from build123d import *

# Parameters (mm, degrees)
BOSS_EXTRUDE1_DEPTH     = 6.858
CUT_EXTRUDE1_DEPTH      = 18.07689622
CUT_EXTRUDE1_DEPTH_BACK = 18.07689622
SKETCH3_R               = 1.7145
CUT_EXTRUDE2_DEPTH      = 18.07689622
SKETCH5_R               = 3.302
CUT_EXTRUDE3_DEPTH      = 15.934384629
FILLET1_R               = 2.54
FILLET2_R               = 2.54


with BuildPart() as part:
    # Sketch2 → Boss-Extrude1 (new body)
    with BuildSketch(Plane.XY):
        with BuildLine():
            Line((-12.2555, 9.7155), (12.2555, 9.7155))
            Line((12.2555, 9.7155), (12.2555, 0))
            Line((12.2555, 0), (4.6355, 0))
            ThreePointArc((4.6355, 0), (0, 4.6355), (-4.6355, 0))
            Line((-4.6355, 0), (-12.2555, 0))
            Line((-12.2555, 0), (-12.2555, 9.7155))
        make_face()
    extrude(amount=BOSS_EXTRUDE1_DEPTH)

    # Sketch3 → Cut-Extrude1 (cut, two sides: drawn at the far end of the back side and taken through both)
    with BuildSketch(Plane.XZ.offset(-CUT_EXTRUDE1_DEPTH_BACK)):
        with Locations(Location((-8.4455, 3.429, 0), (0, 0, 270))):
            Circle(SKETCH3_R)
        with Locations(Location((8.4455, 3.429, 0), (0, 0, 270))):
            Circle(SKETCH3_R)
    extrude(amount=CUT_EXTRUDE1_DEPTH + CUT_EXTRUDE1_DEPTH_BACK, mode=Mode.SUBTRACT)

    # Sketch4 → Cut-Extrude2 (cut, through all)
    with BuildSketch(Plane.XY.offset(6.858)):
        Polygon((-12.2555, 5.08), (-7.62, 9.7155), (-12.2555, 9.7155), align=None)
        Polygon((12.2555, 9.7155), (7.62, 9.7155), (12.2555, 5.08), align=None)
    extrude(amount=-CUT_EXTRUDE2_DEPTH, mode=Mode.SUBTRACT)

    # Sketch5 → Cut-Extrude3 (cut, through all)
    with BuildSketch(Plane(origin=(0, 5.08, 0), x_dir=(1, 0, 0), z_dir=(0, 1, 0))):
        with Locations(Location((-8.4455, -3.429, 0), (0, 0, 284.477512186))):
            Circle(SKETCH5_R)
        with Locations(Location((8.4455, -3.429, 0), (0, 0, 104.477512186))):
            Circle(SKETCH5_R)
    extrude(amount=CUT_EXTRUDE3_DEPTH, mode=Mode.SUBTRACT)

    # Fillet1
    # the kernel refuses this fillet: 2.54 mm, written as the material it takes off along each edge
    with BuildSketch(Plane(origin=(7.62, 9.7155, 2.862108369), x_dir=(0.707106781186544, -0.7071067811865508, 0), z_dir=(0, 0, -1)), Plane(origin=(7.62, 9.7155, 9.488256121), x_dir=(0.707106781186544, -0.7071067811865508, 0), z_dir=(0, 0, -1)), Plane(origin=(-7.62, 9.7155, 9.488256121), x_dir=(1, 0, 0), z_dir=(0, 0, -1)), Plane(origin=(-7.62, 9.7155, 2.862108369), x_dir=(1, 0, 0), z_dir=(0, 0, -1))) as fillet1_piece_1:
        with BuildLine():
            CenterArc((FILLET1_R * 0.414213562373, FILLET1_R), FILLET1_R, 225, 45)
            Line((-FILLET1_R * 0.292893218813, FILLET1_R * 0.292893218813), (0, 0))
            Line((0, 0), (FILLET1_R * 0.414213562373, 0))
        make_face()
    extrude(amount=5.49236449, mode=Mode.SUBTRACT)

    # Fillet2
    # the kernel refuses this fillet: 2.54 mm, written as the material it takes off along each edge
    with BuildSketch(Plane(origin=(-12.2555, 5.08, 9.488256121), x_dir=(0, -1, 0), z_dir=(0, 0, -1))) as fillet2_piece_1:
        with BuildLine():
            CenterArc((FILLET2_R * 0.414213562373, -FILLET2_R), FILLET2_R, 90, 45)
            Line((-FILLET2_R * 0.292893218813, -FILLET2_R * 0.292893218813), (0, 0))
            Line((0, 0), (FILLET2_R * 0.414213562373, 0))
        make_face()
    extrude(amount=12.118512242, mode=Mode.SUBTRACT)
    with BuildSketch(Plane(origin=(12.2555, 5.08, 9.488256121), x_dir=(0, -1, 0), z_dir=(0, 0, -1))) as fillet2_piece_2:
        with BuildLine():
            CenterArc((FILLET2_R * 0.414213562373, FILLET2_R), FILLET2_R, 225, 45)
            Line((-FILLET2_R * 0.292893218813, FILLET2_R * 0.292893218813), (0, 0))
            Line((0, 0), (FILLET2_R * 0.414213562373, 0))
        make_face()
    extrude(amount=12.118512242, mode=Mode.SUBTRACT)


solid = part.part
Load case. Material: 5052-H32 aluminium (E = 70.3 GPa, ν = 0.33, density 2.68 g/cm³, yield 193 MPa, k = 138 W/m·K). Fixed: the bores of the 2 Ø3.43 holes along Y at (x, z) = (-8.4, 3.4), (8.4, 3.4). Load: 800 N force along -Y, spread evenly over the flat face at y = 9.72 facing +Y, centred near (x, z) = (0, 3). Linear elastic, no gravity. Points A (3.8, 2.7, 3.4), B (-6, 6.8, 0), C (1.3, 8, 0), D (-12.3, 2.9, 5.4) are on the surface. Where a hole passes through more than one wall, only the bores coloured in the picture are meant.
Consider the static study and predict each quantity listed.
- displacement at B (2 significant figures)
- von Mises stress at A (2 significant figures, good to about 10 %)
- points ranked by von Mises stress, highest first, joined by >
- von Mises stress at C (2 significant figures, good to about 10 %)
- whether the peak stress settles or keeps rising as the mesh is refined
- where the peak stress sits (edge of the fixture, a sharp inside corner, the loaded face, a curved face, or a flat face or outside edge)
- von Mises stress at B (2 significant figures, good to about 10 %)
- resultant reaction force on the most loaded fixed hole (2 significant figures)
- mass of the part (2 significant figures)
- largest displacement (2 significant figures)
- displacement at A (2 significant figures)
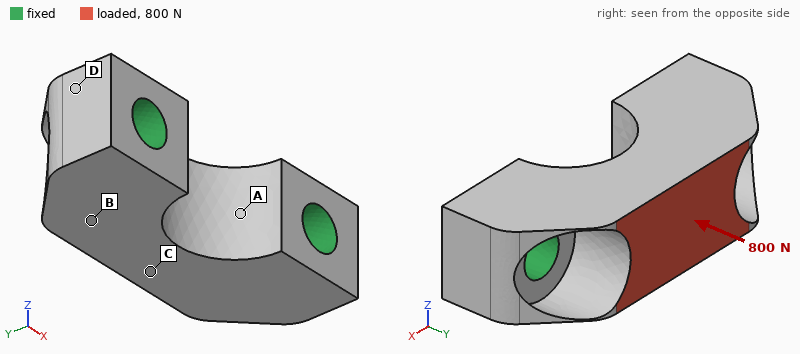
1.6 µm
21 MPa
A > B > C > D
9.7 MPa
keeps rising
edge of the fixture
16 MPa
460 N
2.5 g
3.1 µm
1.6 µm
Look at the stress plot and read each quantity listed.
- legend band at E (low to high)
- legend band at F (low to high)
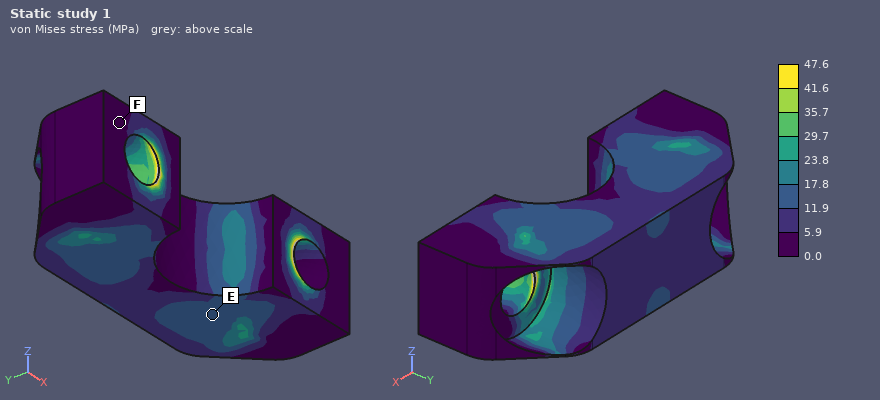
11.9 to 17.8 MPa
0.0 to 5.9 MPa
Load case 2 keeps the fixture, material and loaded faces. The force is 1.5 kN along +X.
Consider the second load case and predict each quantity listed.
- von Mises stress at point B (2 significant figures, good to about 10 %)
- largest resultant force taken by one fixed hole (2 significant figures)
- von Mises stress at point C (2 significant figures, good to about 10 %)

39 MPa
1.0 kN
45 MPa
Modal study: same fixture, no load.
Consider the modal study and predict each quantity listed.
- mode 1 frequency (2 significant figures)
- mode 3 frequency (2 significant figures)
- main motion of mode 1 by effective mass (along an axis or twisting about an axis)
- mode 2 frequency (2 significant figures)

40 kHz
80 kHz
along Z
80 kHz
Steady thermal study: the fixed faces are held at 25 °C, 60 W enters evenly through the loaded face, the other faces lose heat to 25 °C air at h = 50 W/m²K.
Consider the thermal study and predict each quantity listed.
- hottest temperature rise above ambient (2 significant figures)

59 K
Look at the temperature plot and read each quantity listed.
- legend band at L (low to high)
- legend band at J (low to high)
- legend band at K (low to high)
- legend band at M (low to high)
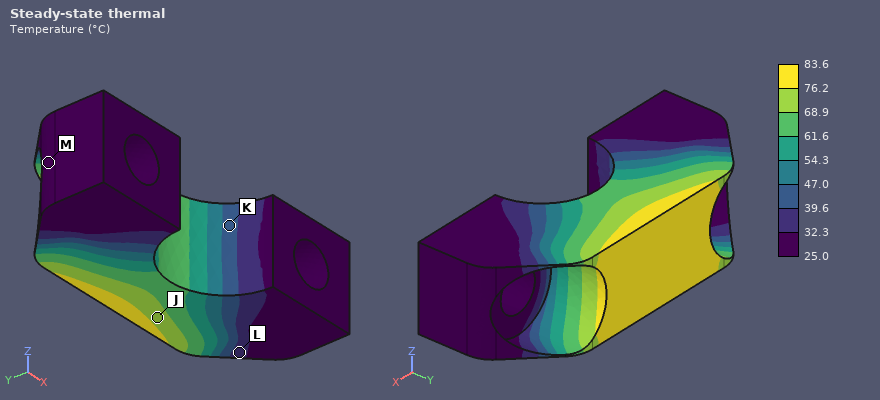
32.3 to 39.6 °C
68.9 to 76.2 °C
39.6 to 47.0 °C
25.0 to 32.3 °C
